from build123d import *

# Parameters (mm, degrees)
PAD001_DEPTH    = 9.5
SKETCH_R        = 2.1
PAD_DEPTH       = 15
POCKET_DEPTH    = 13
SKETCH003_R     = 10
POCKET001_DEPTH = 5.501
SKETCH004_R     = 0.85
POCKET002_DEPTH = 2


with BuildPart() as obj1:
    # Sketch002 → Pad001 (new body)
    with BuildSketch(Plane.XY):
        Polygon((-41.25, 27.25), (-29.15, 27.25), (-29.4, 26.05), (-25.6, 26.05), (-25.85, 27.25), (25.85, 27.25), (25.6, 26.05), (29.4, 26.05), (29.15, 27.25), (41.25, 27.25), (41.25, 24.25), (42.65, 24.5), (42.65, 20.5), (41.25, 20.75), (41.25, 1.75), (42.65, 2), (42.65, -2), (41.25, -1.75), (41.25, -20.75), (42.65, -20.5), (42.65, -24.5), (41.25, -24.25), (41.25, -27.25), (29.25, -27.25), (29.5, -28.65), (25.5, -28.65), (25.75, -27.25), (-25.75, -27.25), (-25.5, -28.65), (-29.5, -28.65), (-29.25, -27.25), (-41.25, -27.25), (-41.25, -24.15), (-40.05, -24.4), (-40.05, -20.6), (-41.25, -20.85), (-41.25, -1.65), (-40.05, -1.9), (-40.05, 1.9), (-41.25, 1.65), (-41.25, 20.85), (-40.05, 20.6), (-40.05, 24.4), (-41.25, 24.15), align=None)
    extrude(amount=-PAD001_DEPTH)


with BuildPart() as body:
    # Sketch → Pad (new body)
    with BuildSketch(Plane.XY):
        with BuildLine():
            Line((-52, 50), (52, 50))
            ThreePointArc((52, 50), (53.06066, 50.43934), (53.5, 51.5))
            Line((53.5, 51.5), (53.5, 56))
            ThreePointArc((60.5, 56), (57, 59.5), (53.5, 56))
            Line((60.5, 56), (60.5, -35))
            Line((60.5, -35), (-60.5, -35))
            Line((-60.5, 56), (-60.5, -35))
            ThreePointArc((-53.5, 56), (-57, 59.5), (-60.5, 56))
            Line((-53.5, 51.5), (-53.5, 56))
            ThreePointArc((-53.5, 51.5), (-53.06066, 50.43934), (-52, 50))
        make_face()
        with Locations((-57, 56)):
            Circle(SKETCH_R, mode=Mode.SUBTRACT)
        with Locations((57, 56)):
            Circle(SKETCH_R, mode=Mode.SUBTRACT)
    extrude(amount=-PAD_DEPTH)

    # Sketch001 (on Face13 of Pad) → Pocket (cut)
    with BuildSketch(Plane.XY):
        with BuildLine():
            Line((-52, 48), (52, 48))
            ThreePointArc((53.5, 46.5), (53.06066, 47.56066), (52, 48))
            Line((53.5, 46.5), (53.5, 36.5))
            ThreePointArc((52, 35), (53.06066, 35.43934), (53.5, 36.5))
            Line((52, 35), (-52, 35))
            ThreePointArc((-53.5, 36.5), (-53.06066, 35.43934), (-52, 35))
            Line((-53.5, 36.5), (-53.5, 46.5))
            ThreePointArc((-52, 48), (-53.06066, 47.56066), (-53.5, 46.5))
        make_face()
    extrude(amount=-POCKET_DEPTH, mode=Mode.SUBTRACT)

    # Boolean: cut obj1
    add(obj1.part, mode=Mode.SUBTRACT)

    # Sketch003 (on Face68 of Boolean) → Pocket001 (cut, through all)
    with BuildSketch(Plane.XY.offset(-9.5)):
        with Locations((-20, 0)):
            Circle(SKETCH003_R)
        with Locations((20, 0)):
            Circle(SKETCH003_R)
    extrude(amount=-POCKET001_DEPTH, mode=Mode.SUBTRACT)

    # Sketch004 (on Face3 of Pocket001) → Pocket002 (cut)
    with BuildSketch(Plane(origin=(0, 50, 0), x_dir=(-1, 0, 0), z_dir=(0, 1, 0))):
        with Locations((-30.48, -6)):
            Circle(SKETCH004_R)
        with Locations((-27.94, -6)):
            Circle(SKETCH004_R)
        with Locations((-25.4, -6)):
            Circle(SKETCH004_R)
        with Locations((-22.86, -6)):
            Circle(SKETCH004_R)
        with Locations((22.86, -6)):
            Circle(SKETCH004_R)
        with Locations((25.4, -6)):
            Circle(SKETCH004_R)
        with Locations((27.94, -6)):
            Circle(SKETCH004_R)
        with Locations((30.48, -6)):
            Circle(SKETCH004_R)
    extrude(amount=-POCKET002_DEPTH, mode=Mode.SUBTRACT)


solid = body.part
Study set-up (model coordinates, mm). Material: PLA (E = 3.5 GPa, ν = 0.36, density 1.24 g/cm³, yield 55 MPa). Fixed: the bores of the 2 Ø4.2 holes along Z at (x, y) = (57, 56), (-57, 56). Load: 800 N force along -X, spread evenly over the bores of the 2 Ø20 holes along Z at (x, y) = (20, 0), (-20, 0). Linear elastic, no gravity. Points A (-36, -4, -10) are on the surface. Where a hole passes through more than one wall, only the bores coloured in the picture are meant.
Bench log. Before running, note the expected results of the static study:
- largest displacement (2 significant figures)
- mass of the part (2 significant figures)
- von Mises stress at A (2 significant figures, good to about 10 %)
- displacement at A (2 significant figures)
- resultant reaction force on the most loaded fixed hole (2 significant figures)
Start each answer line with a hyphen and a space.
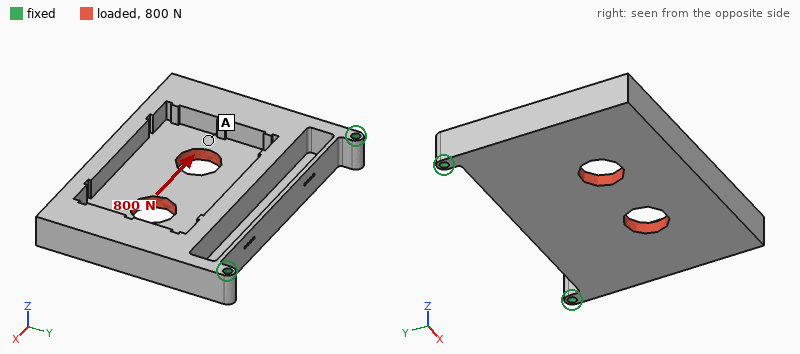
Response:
- 0.23 mm
- 110 g
- 2.4 MPa
- 0.18 mm
- 530 N
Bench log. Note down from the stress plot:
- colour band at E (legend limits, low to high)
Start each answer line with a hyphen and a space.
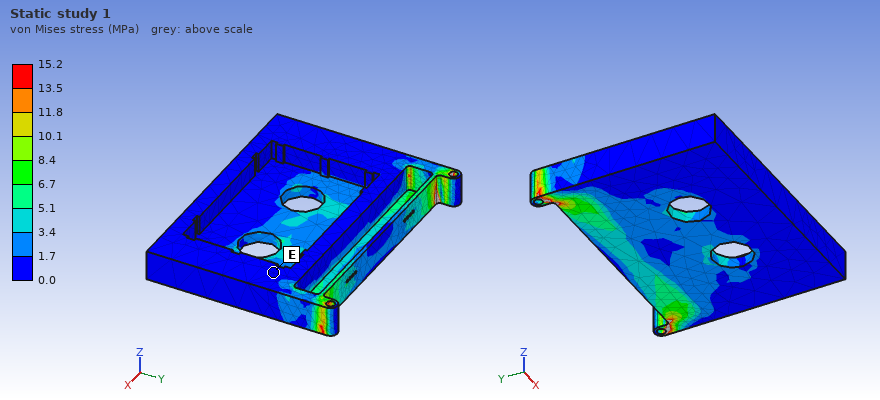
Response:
- 0.0 to 1.7 MPa
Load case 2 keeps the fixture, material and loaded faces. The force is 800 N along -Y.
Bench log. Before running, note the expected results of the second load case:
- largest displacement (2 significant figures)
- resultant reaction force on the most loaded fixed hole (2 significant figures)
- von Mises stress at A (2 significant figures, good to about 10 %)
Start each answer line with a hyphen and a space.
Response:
- 0.47 mm
- 410 N
- 2.6 MPa
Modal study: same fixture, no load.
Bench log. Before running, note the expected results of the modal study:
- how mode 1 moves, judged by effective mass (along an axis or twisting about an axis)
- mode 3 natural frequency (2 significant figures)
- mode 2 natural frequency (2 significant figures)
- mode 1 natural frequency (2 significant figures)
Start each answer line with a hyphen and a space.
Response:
- along Z
- 1000 Hz
- 490 Hz
- 240 Hz
